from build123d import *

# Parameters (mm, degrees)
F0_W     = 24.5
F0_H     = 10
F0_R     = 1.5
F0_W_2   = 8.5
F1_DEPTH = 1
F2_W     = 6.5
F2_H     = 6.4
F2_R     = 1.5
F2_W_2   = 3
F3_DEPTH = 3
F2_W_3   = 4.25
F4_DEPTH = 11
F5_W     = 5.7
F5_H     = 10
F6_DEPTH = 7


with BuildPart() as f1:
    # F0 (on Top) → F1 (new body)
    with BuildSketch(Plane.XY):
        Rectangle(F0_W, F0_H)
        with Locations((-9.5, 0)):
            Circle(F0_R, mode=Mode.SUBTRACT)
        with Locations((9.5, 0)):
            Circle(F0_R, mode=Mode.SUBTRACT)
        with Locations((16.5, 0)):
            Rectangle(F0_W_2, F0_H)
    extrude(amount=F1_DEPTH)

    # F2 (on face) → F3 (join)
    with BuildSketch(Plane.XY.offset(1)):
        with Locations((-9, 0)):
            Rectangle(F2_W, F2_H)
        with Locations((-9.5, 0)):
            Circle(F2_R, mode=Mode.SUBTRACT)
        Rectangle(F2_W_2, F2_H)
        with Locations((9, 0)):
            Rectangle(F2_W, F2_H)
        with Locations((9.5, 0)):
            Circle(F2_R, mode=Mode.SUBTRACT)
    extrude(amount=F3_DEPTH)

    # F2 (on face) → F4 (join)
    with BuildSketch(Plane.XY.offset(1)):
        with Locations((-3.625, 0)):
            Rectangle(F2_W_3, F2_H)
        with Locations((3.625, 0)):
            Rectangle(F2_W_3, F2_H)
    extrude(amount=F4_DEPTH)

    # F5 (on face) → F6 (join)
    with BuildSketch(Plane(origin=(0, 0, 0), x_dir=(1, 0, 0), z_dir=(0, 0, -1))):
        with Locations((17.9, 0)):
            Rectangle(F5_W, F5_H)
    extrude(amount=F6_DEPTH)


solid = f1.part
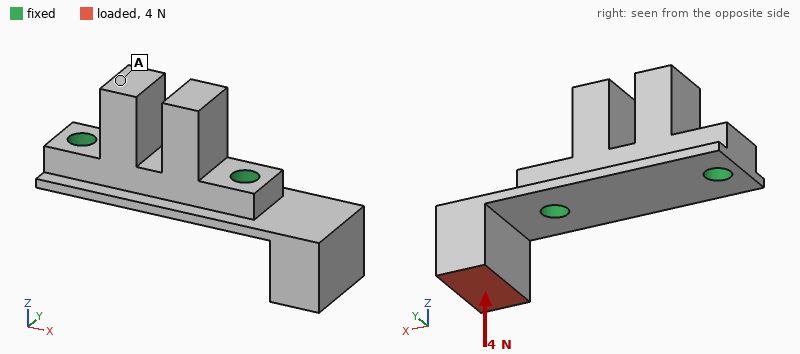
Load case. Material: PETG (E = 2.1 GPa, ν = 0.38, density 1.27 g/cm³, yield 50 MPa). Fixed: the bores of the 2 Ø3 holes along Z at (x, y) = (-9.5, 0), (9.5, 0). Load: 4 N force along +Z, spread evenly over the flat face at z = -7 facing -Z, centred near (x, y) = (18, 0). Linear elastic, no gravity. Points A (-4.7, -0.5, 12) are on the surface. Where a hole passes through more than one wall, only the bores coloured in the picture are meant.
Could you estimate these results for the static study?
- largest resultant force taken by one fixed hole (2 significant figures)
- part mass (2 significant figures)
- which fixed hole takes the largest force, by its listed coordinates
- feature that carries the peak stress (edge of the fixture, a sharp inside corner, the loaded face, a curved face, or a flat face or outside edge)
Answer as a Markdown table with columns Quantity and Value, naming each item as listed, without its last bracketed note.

| Quantity | Value |
|---|---|
| largest resultant force taken by one fixed hole | 4.1 N |
| part mass | 2.0 g |
| which fixed hole takes the largest force, by its listed coordinates | (9.5, 0) |
| feature that carries the peak stress | a flat face or outside edge |
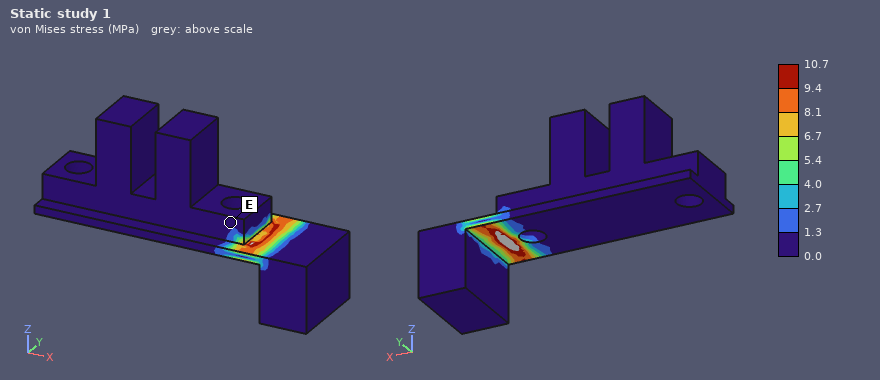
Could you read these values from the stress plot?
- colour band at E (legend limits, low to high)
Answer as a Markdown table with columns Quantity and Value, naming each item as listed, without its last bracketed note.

| Quantity | Value |
|---|---|
| colour band at E | 0.0 to 1.3 MPa |
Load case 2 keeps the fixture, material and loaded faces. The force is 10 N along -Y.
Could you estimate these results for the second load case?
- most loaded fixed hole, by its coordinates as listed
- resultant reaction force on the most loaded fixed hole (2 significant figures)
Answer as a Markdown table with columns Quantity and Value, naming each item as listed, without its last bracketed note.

| Quantity | Value |
|---|---|
| most loaded fixed hole, by its coordinates as listed | (9.5, 0) |
| resultant reaction force on the most loaded fixed hole | 12 N |
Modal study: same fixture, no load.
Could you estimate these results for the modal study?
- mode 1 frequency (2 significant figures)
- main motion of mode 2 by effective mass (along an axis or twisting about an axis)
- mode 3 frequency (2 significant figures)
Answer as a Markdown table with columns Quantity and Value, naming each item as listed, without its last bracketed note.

| Quantity | Value |
|---|---|
| mode 1 frequency | 730 Hz |
| main motion of mode 2 by effective mass | along Y |
| mode 3 frequency | 4900 Hz |
